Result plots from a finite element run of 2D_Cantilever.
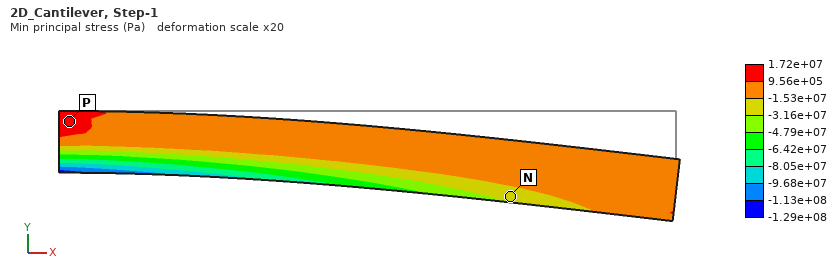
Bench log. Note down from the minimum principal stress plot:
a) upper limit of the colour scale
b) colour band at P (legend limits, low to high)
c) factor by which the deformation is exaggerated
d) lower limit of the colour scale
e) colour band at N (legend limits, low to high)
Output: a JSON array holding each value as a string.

["1.72e+07 Pa", "9.56e+05 to 1.72e+07 Pa", "20", "-1.29e+08 Pa", "-3.16e+07 to -1.53e+07 Pa"]
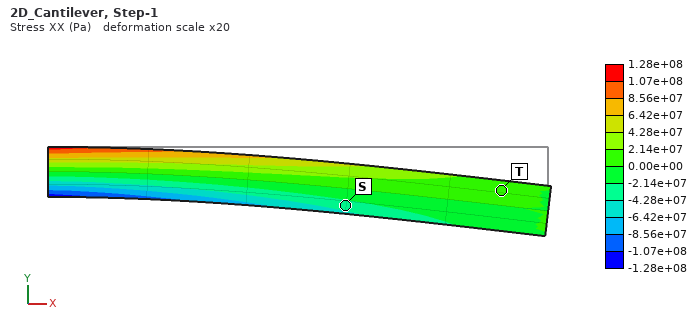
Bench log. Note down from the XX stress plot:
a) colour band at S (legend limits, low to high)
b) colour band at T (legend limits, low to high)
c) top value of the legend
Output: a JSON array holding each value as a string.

["-4.28e+07 to -2.14e+07 Pa", "0.00e+00 to 2.14e+07 Pa", "1.28e+08 Pa"]
